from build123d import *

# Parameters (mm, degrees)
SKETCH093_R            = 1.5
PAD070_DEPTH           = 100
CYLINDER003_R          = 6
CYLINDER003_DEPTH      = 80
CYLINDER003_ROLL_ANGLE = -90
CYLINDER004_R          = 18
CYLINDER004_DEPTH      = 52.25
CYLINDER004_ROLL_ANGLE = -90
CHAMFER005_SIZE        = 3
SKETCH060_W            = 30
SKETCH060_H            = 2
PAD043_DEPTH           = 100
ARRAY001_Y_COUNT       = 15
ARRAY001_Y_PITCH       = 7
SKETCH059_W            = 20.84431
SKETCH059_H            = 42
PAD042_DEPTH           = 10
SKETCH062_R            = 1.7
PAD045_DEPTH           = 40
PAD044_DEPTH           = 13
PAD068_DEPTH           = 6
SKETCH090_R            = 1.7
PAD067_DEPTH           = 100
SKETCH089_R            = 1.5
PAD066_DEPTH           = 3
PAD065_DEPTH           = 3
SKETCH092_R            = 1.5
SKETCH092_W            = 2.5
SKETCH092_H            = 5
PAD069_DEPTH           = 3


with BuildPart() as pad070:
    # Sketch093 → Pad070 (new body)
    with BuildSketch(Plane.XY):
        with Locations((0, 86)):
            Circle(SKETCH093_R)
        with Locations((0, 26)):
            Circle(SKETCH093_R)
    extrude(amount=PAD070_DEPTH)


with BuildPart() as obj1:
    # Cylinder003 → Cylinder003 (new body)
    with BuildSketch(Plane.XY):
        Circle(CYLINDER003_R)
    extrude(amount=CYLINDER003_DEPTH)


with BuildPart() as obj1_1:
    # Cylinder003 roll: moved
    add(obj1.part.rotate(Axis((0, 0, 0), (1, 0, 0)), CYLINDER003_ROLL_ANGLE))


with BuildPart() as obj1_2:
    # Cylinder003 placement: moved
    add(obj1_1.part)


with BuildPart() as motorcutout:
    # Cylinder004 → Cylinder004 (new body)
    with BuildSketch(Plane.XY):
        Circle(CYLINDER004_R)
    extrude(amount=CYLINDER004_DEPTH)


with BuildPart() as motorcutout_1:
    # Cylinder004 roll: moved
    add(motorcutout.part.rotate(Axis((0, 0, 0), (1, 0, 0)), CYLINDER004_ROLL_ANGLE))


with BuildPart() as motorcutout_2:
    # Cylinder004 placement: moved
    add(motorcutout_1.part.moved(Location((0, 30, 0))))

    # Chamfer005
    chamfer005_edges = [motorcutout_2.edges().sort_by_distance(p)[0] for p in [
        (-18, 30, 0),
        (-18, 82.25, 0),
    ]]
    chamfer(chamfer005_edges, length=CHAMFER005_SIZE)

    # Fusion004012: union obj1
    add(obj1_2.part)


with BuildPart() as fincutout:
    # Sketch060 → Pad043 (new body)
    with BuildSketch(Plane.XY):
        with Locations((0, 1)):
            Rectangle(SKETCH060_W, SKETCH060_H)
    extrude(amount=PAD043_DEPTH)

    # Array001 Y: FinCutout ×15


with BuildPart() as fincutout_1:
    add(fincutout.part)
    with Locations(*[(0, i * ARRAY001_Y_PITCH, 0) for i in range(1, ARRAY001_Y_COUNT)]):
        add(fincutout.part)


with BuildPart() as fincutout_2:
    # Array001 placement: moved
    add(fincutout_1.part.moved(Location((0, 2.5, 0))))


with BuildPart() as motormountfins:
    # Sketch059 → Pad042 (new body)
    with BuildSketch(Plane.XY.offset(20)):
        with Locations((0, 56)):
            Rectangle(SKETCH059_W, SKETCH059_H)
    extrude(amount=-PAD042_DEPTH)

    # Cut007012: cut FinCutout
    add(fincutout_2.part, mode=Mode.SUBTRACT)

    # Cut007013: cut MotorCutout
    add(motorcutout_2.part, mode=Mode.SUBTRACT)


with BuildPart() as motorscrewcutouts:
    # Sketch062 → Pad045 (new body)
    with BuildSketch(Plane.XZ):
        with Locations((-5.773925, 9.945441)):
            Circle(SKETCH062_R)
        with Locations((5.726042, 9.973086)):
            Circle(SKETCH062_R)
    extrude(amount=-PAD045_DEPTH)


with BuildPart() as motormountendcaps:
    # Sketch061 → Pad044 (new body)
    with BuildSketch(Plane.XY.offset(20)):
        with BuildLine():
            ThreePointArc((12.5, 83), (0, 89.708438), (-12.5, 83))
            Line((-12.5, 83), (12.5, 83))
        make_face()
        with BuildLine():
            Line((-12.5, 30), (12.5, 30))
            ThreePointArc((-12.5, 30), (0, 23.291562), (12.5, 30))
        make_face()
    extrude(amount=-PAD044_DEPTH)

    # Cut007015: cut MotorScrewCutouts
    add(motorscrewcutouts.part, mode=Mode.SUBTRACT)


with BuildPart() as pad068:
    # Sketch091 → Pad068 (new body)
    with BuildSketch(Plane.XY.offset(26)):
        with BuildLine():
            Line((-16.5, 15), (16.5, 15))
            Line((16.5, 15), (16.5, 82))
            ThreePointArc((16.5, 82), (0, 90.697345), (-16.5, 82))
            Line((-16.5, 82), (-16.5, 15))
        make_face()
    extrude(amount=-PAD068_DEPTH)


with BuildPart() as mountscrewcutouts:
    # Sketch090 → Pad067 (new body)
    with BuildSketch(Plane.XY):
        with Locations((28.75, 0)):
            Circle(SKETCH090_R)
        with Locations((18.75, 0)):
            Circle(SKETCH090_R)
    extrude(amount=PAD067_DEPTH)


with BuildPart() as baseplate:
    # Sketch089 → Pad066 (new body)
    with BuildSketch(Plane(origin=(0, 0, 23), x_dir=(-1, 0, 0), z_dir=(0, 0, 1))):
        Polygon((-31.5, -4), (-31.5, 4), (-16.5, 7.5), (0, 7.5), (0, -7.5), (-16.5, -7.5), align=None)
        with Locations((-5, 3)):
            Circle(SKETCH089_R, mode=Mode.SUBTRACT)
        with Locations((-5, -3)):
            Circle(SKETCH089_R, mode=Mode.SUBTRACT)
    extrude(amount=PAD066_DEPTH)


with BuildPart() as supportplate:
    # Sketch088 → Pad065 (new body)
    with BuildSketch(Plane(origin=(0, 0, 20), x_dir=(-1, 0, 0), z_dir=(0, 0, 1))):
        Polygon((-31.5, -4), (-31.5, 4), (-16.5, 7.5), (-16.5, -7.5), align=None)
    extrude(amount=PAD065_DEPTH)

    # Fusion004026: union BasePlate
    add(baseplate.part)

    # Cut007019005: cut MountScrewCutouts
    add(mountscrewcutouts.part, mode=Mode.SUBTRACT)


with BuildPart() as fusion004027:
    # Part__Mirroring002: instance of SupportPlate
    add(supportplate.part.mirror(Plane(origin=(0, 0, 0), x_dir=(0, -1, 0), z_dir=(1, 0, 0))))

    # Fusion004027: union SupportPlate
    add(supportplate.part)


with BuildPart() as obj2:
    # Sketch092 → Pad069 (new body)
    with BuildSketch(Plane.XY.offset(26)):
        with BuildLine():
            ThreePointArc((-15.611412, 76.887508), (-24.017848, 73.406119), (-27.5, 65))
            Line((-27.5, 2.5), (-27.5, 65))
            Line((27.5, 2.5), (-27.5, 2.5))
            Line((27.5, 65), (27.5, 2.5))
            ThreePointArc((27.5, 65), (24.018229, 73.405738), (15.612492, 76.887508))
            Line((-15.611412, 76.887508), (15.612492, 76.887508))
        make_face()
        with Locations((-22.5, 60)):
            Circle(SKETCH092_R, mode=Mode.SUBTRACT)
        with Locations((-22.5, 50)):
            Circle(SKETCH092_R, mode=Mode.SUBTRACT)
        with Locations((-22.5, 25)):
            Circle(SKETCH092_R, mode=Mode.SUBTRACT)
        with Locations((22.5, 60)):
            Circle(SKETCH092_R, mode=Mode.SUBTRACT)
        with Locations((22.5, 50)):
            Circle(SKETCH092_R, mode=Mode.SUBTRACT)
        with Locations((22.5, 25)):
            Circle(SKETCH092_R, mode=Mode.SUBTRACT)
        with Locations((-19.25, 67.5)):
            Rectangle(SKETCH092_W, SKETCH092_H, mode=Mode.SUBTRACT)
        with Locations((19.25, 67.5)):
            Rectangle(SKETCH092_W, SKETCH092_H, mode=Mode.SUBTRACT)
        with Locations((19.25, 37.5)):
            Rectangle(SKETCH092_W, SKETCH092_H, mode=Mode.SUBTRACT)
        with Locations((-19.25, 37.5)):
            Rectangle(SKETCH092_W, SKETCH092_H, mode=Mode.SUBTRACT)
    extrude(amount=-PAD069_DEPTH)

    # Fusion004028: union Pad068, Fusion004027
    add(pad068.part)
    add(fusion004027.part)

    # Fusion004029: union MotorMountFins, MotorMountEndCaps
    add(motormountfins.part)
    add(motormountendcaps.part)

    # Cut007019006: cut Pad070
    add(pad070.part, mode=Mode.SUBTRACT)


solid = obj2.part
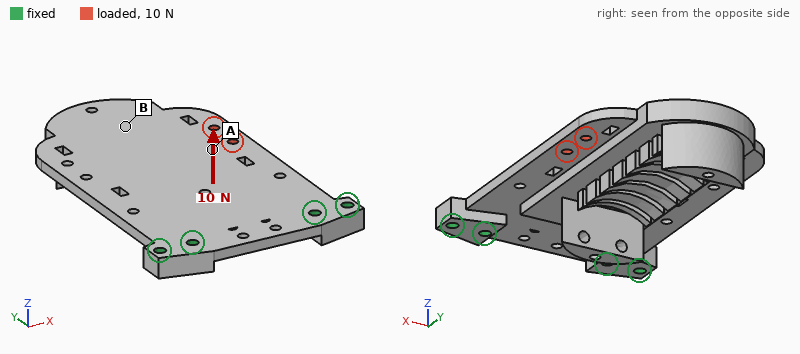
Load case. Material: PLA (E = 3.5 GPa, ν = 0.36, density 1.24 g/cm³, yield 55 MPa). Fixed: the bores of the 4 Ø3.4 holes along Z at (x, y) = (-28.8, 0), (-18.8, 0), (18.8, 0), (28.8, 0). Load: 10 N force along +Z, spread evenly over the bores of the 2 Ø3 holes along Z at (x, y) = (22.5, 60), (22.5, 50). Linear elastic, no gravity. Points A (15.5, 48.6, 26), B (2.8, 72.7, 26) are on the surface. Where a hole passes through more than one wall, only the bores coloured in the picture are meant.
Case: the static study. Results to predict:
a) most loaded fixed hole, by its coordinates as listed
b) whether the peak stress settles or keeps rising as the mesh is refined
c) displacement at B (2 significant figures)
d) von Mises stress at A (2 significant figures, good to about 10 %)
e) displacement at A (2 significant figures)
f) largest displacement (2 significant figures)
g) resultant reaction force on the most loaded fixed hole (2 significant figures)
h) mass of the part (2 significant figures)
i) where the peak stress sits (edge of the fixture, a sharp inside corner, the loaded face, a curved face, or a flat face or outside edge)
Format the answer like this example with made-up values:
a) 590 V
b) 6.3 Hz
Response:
a) (18.8, 0)
b) keeps rising
c) 1.0 mm
d) 0.92 MPa
e) 0.64 mm
f) 1.3 mm
g) 12 N
h) 34 g
i) edge of the fixture
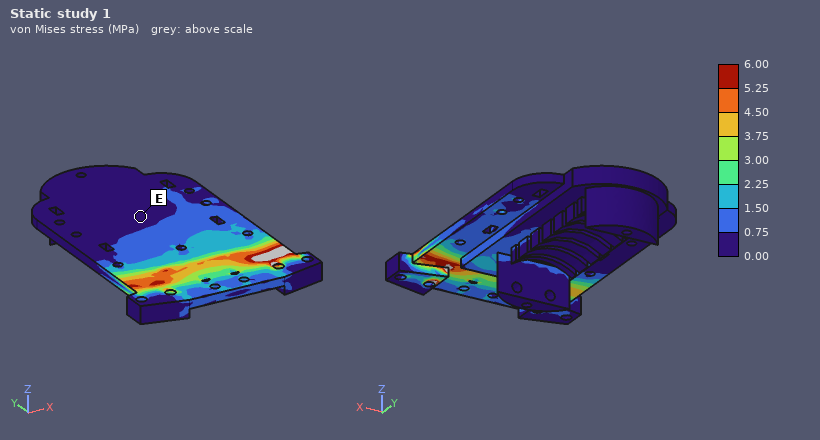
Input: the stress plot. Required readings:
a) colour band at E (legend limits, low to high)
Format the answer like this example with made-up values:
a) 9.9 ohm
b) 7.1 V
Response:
a) 0.00 to 0.75 MPa
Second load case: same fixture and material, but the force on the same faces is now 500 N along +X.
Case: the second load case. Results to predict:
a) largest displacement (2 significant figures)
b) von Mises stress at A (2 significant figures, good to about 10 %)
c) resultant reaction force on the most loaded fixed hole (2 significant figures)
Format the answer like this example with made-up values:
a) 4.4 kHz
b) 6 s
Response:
a) 0.53 mm
b) 10 MPa
c) 370 N
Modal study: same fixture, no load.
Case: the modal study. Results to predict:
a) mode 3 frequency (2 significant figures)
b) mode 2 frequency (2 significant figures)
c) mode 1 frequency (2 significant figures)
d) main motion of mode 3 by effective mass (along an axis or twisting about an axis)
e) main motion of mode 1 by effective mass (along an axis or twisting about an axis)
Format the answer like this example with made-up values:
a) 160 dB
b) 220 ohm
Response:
a) 950 Hz
b) 730 Hz
c) 110 Hz
d) along Z
e) along Z
